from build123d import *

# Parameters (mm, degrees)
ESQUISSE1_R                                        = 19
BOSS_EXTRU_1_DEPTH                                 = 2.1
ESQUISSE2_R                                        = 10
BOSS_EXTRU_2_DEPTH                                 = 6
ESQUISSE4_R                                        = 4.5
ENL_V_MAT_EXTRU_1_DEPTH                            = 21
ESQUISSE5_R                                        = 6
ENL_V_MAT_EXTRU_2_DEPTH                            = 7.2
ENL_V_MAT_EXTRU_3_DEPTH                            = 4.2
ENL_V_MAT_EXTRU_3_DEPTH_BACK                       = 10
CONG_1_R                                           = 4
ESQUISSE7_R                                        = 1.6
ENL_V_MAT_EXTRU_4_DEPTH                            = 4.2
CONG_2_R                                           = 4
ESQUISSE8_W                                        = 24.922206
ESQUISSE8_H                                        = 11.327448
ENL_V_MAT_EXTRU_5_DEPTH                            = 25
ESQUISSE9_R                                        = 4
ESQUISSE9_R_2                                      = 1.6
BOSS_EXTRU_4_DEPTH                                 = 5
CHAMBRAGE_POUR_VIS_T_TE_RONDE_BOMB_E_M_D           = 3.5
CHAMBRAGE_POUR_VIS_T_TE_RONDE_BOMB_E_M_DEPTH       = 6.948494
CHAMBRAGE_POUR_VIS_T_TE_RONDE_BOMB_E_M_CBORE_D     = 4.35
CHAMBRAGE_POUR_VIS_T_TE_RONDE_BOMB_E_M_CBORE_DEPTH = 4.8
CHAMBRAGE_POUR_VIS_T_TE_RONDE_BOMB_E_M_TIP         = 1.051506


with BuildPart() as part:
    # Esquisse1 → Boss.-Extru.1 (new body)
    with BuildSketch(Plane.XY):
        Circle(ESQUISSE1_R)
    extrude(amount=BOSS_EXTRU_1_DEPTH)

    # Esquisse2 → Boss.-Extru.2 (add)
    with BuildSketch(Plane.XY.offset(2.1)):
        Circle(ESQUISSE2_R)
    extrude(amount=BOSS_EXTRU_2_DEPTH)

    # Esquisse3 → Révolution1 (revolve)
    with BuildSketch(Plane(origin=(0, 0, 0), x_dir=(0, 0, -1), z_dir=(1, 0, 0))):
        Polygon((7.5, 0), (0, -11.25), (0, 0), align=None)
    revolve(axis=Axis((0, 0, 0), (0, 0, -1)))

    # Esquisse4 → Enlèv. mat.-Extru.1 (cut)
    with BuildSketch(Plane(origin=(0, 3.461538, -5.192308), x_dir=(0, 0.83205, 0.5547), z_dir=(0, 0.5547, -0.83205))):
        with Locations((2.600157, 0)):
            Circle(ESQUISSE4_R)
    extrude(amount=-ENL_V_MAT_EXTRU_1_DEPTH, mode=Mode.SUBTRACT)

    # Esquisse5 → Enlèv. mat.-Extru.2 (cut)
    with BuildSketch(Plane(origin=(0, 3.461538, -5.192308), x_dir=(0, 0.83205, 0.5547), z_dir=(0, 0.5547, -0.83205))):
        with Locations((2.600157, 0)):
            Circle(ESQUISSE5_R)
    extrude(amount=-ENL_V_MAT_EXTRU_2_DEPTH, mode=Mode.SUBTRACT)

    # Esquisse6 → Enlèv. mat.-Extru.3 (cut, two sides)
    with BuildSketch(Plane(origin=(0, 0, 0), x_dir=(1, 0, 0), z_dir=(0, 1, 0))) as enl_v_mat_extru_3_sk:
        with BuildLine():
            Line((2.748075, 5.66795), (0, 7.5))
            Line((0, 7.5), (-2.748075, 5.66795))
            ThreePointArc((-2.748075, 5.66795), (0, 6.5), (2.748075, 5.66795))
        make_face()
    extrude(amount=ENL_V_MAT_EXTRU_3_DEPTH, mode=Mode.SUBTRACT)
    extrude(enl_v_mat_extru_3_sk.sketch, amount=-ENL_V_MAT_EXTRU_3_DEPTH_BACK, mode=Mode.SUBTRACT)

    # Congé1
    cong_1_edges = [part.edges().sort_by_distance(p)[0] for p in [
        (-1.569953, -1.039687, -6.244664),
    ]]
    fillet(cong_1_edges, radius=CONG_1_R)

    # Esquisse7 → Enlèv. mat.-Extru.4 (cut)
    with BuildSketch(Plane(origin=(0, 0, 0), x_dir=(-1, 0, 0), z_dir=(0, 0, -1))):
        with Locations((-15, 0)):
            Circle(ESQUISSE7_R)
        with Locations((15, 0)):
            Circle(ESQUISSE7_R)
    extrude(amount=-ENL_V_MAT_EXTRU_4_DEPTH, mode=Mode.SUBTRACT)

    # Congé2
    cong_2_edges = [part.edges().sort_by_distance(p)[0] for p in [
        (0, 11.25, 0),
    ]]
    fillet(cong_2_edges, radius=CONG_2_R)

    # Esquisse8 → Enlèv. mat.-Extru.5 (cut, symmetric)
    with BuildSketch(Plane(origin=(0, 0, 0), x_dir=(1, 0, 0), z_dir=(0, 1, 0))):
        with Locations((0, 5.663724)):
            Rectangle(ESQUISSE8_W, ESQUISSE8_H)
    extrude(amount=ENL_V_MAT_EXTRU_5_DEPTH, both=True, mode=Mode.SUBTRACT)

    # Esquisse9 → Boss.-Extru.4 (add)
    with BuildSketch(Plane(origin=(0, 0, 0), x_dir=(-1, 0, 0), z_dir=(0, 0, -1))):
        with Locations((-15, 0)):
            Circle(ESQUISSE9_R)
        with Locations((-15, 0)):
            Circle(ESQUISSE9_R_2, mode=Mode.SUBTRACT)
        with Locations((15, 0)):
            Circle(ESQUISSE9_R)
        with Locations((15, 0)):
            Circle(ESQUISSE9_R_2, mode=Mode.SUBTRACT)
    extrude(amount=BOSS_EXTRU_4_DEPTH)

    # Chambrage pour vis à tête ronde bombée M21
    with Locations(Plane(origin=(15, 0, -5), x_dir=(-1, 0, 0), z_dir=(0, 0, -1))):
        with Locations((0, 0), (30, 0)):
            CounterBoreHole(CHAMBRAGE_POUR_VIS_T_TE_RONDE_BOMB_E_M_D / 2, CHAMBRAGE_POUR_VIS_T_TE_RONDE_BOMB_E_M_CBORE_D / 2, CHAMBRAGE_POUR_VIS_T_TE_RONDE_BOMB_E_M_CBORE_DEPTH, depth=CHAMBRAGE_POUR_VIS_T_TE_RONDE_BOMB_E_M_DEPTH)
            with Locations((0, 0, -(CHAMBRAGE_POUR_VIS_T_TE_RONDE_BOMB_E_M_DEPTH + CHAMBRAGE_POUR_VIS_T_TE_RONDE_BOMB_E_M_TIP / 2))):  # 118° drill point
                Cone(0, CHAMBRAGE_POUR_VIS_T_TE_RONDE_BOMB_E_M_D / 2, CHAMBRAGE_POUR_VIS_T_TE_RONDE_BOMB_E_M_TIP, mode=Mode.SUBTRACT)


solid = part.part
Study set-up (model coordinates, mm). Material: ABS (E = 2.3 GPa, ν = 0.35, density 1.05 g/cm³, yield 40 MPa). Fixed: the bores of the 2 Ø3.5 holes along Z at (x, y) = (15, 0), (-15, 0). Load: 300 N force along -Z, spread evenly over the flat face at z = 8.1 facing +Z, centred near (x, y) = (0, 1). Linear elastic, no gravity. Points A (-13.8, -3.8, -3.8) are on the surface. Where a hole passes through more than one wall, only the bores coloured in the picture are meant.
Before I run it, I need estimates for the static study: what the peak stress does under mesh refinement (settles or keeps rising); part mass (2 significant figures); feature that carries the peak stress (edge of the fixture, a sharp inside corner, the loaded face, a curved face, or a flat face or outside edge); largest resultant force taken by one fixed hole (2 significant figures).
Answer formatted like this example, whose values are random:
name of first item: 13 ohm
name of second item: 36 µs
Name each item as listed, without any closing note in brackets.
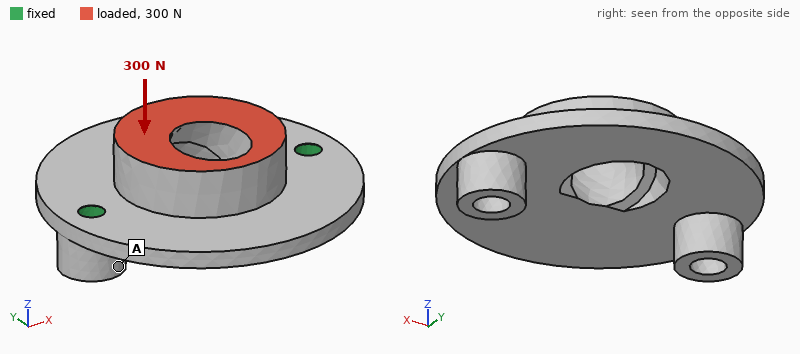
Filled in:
what the peak stress does under mesh refinement: keeps rising
part mass: 4.0 g
feature that carries the peak stress: edge of the fixture
largest resultant force taken by one fixed hole: 190 N
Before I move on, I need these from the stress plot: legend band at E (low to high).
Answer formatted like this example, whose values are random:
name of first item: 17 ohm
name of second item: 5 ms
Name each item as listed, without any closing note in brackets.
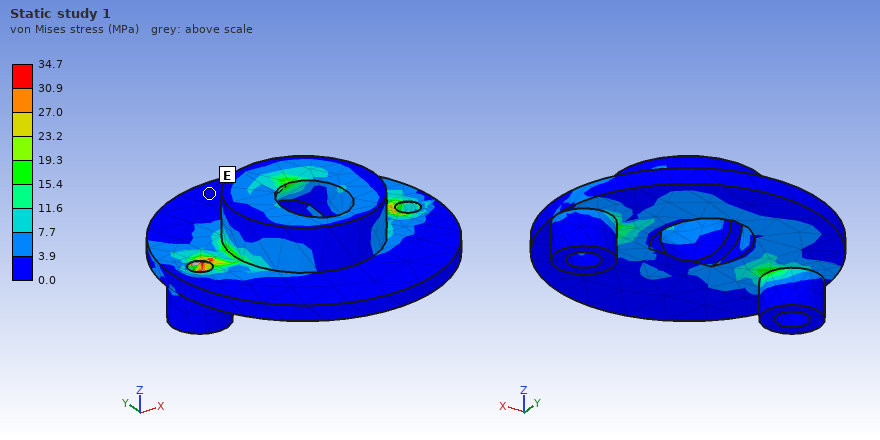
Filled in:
legend band at E: 0.0 to 3.9 MPa
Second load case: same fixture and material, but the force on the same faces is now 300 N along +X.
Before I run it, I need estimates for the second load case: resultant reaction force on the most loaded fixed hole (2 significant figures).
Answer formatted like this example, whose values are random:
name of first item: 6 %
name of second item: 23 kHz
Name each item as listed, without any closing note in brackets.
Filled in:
resultant reaction force on the most loaded fixed hole: 180 N
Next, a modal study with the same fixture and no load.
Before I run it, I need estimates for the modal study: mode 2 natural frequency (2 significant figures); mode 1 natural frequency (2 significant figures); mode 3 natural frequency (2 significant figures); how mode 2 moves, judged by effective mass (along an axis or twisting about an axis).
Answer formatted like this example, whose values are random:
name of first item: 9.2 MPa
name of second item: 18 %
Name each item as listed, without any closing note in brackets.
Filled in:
mode 2 natural frequency: 3200 Hz
mode 1 natural frequency: 1700 Hz
mode 3 natural frequency: 5200 Hz
how mode 2 moves, judged by effective mass: along Z
